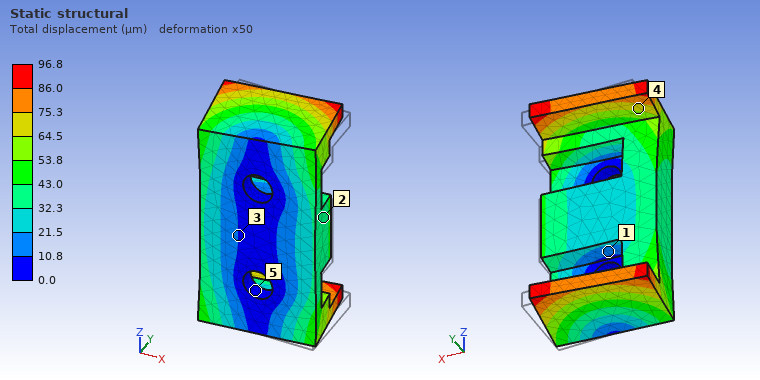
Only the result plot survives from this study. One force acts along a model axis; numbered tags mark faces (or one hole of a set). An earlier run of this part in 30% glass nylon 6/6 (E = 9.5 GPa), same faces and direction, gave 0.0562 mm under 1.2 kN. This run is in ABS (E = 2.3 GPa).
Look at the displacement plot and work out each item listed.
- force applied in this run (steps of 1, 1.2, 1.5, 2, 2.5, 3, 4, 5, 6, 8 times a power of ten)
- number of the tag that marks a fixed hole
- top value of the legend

500 N
5
96.8 µm
